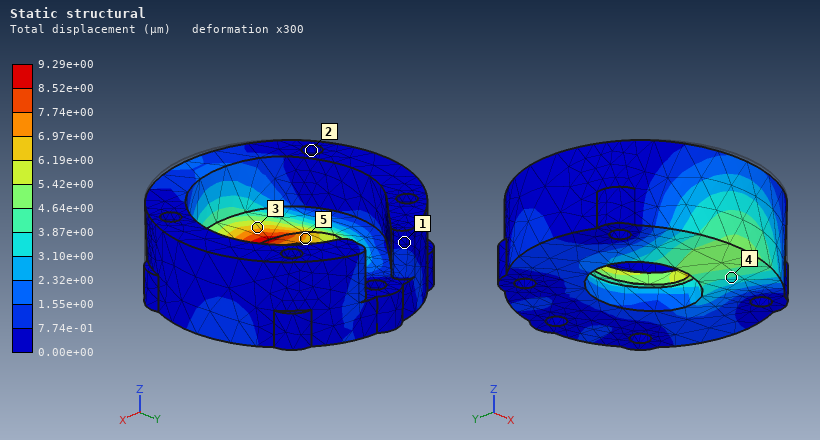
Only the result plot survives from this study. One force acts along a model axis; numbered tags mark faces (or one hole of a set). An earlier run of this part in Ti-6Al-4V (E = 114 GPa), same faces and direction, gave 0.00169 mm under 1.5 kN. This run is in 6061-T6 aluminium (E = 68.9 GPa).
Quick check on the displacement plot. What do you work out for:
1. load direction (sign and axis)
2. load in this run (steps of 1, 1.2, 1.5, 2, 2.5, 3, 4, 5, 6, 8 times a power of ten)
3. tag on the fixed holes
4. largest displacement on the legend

+Y
5 kN
2
9.29e+00 µm
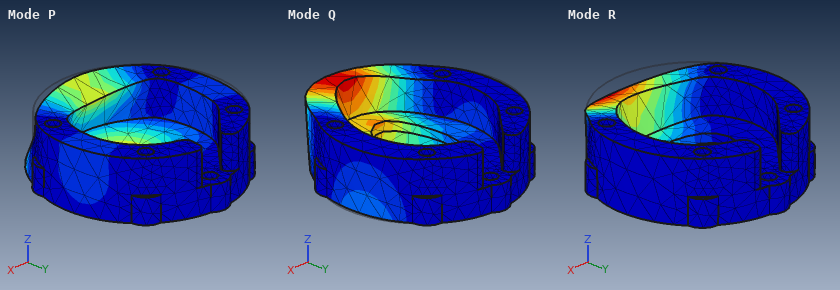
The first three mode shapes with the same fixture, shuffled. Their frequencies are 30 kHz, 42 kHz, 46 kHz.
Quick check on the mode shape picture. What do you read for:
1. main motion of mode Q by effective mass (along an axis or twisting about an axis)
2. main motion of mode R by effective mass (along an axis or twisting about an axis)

along Y
along Z
